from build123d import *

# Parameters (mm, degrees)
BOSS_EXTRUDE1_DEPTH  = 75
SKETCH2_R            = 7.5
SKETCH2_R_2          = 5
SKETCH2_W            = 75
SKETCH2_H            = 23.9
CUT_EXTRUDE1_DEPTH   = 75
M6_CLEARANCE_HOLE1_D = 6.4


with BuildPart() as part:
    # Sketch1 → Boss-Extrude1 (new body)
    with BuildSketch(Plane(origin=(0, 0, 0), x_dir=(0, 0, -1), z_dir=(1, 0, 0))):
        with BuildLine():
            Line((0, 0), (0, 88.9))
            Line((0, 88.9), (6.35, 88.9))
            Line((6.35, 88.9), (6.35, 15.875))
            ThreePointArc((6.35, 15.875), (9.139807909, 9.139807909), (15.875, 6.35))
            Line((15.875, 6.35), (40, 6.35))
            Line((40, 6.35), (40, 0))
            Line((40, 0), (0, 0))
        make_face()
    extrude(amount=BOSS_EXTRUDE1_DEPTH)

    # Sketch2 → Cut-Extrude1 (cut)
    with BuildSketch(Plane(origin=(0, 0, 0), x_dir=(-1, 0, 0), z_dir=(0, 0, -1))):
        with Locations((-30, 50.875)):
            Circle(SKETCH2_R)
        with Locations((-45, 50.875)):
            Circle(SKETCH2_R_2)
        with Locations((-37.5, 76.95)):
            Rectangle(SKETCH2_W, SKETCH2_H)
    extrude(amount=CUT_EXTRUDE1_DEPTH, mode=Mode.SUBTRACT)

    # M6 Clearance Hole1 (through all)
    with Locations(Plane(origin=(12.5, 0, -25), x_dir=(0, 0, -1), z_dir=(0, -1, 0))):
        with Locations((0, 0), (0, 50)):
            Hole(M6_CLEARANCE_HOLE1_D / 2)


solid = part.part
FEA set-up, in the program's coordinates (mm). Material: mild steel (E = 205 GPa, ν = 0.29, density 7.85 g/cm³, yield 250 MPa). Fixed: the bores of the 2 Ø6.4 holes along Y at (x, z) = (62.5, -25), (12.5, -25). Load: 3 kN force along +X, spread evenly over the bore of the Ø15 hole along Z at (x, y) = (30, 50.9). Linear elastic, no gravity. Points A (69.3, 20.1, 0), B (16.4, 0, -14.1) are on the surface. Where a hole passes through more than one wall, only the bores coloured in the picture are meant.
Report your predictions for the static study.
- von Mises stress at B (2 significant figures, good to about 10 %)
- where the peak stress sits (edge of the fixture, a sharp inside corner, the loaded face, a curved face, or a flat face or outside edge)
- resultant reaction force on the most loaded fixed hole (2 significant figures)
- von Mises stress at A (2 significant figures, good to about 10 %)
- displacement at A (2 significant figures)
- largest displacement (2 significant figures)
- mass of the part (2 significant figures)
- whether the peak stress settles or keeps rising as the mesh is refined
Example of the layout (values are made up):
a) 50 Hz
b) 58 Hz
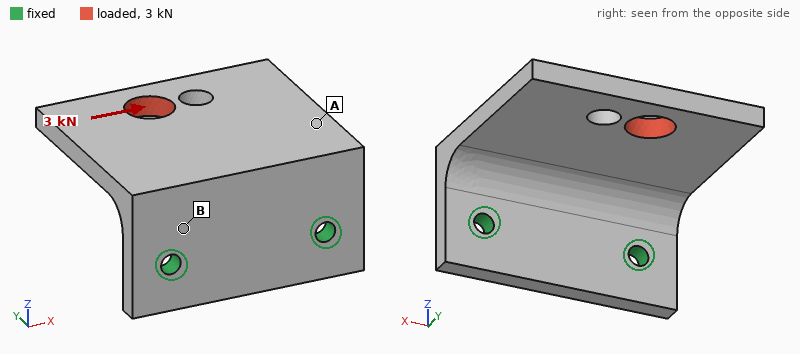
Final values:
a) 53 MPa
b) edge of the fixture
c) 3.3 kN
d) 25 MPa
e) 46 µm
f) 99 µm
g) 360 g
h) keeps rising
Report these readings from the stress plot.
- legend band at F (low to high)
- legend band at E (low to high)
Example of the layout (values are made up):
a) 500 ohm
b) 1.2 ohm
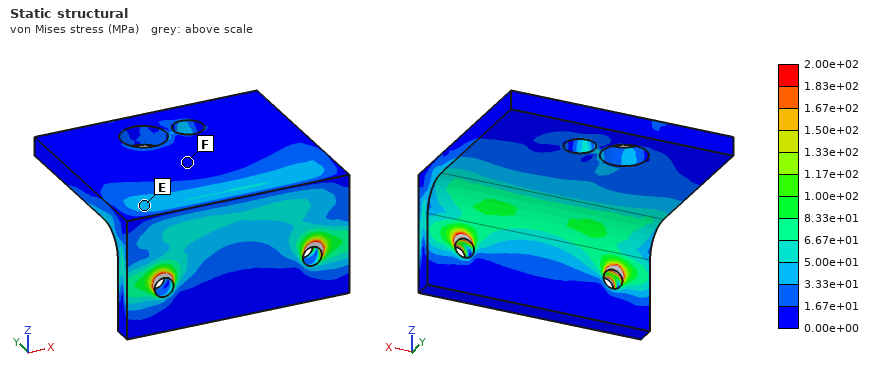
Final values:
a) 0.00e+00 to 1.67e+01 MPa
b) 3.33e+01 to 5.00e+01 MPa
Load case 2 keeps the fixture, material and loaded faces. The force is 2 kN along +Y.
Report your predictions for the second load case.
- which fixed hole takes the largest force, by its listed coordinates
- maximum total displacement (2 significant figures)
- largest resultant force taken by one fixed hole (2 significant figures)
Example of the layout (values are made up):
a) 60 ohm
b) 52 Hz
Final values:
a) (12.5, -25)
b) 0.10 mm
c) 1.3 kN
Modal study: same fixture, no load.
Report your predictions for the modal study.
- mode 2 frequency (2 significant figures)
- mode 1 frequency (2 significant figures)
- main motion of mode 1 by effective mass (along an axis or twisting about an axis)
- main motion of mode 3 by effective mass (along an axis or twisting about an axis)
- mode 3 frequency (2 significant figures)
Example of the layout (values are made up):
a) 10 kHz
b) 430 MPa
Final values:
a) 2300 Hz
b) 1100 Hz
c) along Z
d) along X
e) 3500 Hz
